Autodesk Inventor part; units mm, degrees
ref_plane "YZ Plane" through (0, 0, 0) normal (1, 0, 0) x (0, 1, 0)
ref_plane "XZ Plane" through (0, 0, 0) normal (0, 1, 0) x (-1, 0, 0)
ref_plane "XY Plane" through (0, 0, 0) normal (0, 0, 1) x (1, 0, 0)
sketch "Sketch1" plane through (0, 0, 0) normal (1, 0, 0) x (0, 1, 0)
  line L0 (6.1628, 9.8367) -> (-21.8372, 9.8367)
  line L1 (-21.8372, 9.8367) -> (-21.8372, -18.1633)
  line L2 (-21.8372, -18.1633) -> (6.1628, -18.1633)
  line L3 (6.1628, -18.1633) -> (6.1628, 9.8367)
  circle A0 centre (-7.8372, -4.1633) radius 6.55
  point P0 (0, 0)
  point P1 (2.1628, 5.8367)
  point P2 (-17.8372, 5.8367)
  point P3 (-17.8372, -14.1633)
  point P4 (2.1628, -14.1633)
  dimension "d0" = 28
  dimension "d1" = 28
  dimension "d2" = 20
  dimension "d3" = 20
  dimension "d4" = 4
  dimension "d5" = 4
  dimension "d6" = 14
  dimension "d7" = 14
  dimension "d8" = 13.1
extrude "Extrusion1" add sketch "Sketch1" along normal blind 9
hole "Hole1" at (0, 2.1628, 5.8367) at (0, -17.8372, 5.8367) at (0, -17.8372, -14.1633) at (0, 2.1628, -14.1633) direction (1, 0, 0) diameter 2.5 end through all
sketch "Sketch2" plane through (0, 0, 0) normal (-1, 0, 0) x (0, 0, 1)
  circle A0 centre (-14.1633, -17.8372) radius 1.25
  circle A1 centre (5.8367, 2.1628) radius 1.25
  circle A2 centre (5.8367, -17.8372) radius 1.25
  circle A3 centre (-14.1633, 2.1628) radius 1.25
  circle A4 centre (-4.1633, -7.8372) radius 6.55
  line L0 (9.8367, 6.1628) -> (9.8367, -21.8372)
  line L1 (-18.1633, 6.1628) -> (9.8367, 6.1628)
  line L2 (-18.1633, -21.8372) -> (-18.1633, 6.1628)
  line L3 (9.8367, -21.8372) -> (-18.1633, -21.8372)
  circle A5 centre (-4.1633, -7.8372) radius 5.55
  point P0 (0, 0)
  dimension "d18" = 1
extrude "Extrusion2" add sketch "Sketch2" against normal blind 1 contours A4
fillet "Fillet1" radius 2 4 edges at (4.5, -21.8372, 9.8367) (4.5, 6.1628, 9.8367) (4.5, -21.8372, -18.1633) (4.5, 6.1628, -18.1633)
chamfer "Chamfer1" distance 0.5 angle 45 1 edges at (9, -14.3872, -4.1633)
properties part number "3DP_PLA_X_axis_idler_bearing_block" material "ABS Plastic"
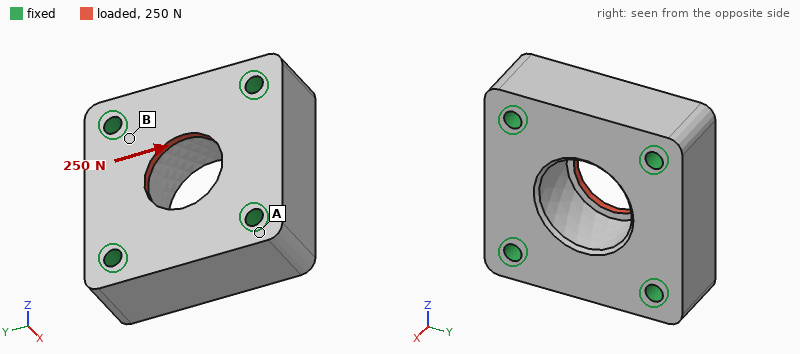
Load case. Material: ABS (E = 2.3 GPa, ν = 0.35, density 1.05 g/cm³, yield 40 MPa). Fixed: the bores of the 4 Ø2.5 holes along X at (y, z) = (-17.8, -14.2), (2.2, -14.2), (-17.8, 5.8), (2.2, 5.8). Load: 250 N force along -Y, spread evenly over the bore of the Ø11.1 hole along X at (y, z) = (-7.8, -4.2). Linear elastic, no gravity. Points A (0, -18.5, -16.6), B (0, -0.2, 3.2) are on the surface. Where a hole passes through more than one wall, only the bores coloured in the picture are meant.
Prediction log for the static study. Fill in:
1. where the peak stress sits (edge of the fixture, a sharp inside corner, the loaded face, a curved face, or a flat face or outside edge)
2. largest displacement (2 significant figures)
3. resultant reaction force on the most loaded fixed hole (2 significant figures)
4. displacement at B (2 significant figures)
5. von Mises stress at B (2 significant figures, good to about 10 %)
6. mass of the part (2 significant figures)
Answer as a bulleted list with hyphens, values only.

- a sharp inside corner
- 25 µm
- 68 N
- 3.7 µm
- 3.0 MPa
- 6.0 g
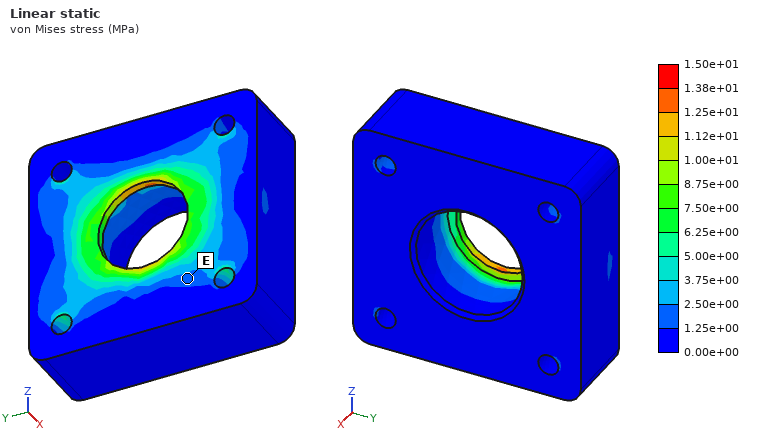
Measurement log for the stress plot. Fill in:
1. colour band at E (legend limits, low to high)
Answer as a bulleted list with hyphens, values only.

- 1.25e+00 to 2.50e+00 MPa
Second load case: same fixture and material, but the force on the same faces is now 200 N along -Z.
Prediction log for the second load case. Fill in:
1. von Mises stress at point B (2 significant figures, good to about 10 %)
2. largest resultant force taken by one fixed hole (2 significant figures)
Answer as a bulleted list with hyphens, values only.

- 2.3 MPa
- 54 N
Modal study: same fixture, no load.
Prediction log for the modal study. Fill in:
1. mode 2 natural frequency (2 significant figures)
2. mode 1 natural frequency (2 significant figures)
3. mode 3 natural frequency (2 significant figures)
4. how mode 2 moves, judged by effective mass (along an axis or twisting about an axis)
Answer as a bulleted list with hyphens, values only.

- 17 kHz
- 14 kHz
- 19 kHz
- along X
